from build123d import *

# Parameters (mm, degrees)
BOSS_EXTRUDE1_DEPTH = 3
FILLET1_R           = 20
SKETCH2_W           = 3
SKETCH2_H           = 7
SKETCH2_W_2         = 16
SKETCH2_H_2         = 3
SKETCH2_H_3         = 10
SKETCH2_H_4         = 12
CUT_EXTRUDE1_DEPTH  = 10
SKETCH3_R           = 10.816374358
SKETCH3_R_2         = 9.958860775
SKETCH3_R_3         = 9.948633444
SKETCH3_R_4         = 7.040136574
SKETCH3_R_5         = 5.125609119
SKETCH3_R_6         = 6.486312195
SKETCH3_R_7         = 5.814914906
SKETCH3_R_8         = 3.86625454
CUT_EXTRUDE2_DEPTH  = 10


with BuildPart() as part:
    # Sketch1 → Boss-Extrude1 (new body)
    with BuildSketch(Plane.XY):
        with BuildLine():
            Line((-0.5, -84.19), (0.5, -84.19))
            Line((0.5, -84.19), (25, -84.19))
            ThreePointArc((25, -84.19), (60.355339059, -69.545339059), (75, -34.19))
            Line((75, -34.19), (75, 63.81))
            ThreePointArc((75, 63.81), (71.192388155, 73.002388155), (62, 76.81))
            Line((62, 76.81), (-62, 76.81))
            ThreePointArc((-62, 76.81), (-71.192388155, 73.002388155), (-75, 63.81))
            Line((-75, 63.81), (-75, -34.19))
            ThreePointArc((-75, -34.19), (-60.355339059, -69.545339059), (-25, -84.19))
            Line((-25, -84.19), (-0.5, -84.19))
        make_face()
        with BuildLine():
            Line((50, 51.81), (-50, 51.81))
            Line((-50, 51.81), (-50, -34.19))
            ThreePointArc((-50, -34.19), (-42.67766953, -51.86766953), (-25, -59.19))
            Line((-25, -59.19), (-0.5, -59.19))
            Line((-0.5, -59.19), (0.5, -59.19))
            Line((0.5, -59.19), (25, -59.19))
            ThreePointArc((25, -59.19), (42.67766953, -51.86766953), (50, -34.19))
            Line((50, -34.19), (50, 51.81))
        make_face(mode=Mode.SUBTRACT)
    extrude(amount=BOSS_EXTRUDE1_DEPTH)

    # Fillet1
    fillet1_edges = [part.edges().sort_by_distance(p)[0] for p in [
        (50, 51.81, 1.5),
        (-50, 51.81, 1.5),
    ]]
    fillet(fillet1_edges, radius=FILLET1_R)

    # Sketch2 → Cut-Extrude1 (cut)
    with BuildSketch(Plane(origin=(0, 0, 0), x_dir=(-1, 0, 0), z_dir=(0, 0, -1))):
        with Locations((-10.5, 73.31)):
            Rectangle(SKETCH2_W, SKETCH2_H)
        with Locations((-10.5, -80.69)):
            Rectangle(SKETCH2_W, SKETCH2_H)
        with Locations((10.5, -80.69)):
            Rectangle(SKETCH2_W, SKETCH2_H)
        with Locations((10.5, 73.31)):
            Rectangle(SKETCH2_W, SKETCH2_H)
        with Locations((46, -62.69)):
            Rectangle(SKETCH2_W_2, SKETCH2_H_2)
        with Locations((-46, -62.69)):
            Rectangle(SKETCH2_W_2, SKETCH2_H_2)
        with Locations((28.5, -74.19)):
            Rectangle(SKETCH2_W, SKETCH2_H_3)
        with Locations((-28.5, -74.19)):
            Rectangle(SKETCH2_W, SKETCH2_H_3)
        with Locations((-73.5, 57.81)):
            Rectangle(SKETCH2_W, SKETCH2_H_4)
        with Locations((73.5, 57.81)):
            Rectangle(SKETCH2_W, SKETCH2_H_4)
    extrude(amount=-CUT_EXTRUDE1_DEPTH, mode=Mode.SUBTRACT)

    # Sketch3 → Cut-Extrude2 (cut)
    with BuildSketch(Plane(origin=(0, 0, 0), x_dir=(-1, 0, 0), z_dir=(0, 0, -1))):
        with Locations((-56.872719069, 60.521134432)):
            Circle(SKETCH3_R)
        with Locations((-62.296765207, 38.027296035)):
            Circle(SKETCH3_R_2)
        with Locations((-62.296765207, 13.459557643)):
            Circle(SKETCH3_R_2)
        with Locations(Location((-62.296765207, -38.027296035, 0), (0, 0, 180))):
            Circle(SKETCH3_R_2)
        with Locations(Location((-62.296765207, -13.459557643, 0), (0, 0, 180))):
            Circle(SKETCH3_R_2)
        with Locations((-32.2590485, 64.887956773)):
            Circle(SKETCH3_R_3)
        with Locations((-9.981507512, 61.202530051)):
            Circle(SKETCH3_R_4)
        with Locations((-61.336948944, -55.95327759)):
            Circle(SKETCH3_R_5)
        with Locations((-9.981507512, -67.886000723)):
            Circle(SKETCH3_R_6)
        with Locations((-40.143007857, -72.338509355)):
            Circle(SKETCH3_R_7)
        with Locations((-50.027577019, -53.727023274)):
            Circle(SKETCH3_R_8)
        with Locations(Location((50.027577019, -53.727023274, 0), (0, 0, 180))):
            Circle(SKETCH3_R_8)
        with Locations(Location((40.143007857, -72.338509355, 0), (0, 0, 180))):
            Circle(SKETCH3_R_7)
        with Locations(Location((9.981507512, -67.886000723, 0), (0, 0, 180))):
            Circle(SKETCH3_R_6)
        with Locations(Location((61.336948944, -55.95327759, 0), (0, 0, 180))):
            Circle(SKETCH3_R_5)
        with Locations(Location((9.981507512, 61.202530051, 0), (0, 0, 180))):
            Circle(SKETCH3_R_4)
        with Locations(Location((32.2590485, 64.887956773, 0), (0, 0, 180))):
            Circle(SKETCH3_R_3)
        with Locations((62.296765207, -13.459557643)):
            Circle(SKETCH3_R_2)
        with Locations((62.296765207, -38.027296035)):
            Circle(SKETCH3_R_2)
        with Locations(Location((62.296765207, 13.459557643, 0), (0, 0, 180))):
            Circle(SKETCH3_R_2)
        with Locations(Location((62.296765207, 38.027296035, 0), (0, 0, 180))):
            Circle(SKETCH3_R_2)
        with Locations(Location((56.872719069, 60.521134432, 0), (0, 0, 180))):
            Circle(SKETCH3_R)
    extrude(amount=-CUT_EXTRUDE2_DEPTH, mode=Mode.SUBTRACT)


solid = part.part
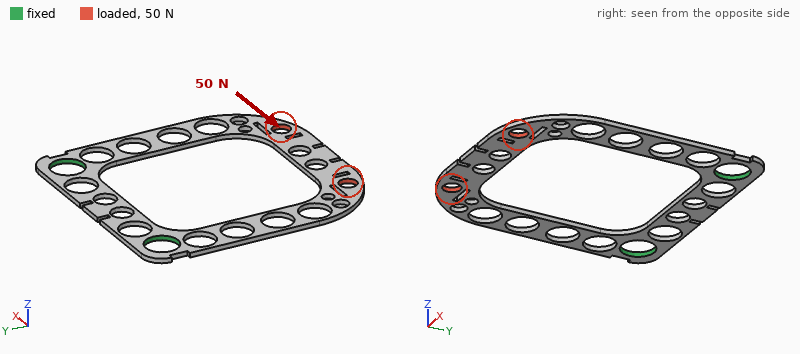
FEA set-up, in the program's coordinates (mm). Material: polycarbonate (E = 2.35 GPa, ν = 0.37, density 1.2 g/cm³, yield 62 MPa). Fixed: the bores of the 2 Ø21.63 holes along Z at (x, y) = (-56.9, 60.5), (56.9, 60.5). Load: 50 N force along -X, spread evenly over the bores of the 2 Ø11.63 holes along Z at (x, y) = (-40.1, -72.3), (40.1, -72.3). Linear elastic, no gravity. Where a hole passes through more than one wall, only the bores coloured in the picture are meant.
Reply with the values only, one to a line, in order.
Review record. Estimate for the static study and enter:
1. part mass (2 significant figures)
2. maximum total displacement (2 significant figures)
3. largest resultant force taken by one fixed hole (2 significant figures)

26 g
1.6 mm
35 N
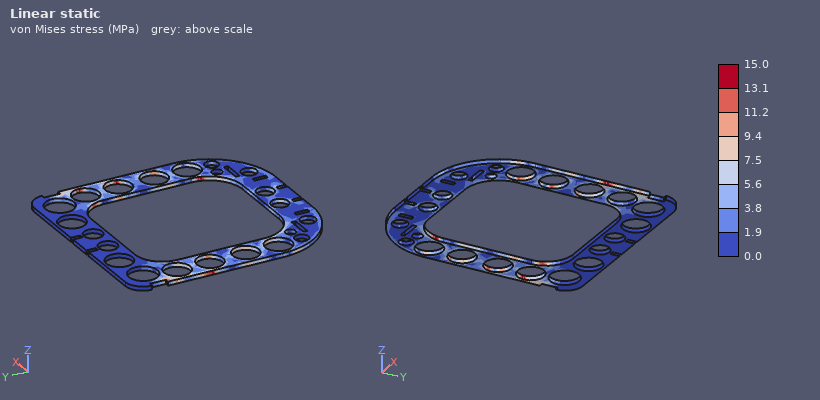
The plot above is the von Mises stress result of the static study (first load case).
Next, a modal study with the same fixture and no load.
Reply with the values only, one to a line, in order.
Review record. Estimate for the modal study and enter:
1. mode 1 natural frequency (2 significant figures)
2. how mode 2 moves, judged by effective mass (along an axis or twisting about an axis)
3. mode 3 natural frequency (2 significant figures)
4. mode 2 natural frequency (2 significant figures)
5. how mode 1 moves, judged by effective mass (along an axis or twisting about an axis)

20 Hz
twisting about Y
150 Hz
58 Hz
along Z
